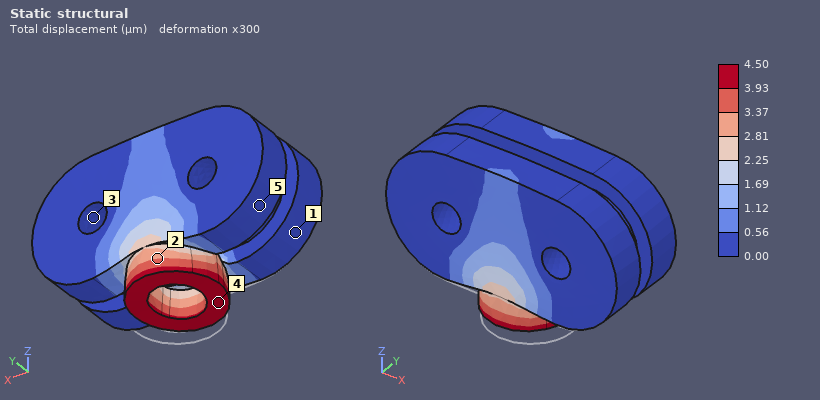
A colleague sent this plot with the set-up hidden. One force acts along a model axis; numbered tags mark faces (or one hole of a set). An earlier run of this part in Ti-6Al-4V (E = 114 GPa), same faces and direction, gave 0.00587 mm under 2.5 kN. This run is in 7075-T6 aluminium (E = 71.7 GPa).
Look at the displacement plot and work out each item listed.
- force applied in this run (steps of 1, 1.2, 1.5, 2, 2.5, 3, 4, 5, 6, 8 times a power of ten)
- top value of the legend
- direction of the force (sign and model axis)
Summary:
1.2 kN
4.50 µm
+Z
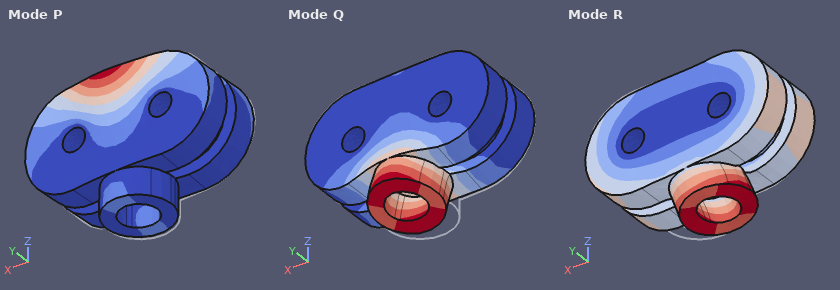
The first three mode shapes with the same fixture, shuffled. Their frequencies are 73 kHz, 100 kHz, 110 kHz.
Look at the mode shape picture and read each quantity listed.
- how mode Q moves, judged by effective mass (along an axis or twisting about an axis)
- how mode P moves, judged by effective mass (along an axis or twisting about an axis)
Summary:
along Y
along Y
